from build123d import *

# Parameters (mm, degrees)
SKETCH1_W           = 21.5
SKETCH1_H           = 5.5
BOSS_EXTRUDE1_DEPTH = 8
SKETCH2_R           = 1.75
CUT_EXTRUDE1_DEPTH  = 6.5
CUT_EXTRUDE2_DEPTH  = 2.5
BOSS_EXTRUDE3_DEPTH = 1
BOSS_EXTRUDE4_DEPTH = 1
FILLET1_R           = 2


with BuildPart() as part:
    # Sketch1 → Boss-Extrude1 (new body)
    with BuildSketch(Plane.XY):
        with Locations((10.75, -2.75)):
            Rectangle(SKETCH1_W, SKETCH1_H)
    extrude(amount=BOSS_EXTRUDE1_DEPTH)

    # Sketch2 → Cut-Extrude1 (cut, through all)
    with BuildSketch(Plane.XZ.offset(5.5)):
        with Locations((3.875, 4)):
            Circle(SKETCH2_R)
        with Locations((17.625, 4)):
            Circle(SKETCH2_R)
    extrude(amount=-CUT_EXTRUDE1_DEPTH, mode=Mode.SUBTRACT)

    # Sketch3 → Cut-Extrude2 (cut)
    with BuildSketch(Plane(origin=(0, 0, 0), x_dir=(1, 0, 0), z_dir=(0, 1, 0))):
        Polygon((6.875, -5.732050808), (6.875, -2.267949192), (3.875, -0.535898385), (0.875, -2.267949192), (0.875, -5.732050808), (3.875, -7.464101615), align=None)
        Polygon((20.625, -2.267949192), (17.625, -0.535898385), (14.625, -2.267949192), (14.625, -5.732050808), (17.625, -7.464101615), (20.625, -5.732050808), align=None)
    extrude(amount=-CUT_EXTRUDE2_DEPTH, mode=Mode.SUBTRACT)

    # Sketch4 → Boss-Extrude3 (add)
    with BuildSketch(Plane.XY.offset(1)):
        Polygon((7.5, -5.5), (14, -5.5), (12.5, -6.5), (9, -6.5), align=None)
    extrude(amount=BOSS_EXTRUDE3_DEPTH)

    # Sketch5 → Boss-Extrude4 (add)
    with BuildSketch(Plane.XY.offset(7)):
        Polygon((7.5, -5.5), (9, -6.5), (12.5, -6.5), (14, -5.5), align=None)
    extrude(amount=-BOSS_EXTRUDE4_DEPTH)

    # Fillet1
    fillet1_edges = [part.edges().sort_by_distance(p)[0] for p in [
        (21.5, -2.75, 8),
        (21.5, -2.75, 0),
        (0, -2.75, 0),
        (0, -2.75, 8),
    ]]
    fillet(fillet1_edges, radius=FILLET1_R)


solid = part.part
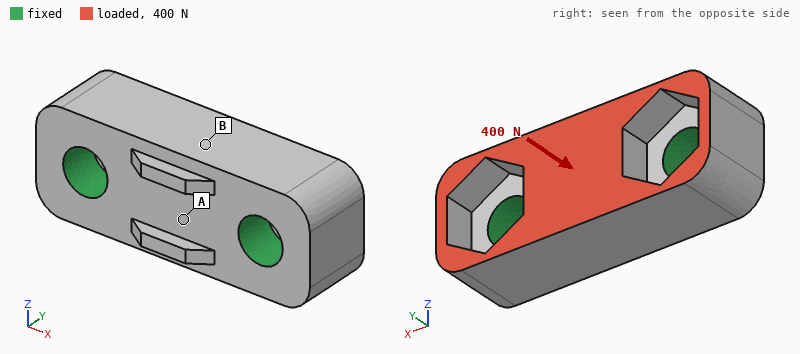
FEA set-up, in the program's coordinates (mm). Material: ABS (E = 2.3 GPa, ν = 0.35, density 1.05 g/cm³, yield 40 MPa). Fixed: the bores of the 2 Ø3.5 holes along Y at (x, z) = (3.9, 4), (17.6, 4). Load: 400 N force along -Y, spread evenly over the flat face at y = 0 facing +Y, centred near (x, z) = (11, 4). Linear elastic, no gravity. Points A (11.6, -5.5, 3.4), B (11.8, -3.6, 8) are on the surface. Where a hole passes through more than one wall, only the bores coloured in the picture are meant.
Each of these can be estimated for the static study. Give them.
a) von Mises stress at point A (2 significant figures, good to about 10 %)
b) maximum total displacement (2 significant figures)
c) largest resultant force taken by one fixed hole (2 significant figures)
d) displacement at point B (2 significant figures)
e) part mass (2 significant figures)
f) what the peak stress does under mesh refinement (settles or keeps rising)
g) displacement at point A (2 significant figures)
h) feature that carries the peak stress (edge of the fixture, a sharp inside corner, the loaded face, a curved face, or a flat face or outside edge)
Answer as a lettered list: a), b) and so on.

a) 5.5 MPa
b) 38 µm
c) 210 N
d) 35 µm
e) 0.76 g
f) keeps rising
g) 30 µm
h) edge of the fixture
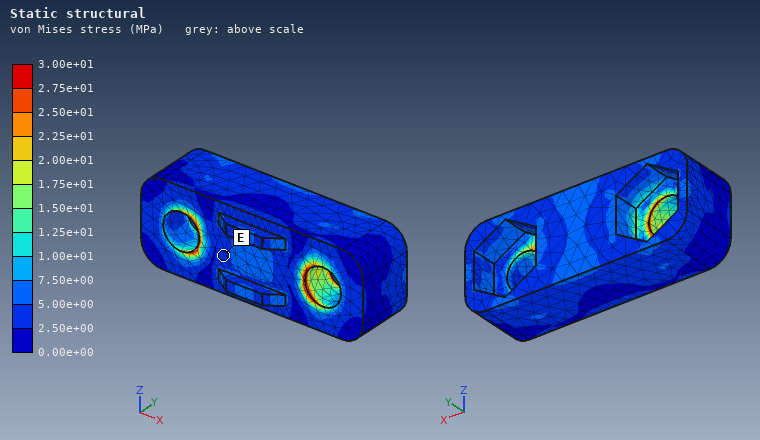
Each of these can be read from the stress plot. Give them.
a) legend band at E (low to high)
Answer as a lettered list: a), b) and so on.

a) 2.50e+00 to 5.00e+00 MPa
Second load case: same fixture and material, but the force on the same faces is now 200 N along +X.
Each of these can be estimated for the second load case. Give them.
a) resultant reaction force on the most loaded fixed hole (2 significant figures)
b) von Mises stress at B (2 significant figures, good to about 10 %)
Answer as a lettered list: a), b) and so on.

a) 110 N
b) 1.7 MPa
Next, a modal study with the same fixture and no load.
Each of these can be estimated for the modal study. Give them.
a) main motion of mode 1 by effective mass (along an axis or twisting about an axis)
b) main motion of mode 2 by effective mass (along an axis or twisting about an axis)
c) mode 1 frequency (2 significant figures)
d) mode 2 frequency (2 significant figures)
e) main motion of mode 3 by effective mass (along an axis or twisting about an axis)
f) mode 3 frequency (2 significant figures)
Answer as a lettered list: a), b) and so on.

a) along Z
b) along Y
c) 18 kHz
d) 23 kHz
e) along Z
f) 27 kHz
